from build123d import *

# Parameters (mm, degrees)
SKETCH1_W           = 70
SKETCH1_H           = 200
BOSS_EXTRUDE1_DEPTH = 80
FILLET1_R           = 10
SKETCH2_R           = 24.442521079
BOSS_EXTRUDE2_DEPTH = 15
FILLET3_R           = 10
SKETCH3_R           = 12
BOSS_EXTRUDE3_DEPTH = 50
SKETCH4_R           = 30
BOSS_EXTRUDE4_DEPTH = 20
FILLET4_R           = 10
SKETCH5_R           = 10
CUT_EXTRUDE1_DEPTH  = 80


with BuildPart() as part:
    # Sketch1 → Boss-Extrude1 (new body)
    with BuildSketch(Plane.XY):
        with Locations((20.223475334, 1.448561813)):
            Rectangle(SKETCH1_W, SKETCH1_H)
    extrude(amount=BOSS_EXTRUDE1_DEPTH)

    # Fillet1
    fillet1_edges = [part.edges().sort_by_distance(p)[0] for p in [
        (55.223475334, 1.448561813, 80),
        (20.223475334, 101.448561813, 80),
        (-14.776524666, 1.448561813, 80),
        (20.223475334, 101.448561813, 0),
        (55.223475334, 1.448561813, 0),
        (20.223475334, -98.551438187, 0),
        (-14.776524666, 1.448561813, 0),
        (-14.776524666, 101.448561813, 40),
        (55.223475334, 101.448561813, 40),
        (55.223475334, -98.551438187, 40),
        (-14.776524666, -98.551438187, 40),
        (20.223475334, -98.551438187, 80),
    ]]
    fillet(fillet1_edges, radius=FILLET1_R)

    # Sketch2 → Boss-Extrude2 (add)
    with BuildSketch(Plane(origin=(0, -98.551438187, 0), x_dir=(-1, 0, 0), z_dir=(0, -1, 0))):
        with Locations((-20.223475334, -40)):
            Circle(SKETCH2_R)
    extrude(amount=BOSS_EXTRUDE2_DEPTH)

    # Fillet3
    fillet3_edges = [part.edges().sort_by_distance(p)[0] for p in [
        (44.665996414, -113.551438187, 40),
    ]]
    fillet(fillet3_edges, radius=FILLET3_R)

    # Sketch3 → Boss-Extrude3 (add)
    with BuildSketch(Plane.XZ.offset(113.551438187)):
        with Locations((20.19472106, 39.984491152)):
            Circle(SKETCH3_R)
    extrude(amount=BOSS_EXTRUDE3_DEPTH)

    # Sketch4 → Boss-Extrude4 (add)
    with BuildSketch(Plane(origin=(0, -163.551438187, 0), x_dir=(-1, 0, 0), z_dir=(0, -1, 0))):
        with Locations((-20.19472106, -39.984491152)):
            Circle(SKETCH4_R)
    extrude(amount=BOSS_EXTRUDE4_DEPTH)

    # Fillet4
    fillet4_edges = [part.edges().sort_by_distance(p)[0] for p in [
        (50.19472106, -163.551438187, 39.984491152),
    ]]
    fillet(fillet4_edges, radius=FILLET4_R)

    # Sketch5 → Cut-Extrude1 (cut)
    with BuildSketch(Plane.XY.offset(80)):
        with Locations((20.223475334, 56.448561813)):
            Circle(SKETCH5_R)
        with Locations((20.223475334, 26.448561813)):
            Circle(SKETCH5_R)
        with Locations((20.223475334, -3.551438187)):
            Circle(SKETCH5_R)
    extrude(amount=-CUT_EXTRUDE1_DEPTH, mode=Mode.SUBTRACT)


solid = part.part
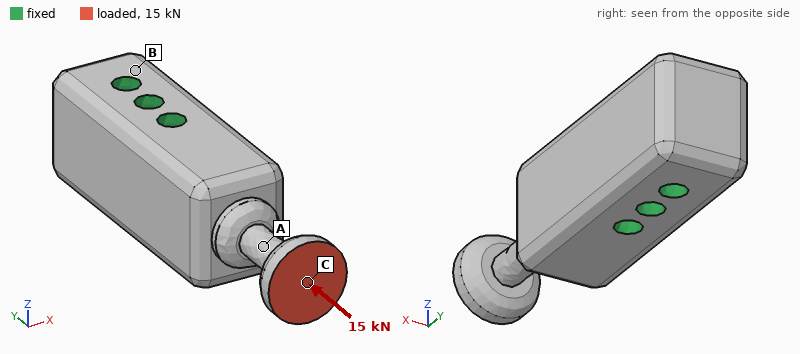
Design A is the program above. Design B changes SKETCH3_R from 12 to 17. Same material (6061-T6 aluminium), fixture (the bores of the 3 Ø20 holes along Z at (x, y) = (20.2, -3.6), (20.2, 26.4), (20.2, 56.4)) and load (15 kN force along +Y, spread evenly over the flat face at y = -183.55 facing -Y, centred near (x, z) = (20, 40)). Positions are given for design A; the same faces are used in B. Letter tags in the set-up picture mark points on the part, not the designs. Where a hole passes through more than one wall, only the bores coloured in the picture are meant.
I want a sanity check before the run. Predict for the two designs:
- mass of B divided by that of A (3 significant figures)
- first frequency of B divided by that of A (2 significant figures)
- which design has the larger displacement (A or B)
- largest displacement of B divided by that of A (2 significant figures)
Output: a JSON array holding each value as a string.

["1.02", "1.4", "A", "0.61"]
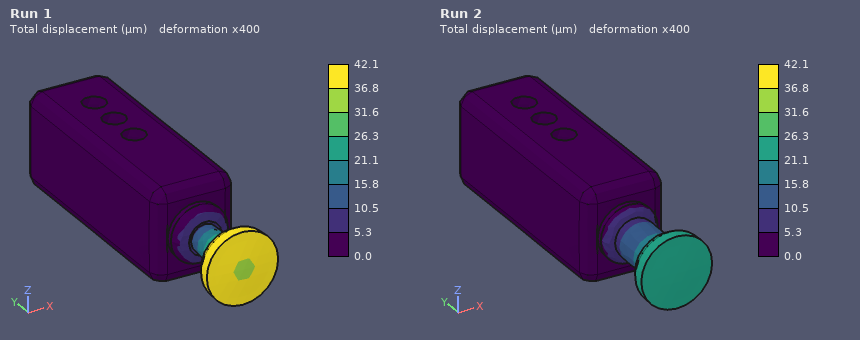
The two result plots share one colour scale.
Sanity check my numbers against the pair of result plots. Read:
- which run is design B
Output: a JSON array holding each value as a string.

["Run 2"]
